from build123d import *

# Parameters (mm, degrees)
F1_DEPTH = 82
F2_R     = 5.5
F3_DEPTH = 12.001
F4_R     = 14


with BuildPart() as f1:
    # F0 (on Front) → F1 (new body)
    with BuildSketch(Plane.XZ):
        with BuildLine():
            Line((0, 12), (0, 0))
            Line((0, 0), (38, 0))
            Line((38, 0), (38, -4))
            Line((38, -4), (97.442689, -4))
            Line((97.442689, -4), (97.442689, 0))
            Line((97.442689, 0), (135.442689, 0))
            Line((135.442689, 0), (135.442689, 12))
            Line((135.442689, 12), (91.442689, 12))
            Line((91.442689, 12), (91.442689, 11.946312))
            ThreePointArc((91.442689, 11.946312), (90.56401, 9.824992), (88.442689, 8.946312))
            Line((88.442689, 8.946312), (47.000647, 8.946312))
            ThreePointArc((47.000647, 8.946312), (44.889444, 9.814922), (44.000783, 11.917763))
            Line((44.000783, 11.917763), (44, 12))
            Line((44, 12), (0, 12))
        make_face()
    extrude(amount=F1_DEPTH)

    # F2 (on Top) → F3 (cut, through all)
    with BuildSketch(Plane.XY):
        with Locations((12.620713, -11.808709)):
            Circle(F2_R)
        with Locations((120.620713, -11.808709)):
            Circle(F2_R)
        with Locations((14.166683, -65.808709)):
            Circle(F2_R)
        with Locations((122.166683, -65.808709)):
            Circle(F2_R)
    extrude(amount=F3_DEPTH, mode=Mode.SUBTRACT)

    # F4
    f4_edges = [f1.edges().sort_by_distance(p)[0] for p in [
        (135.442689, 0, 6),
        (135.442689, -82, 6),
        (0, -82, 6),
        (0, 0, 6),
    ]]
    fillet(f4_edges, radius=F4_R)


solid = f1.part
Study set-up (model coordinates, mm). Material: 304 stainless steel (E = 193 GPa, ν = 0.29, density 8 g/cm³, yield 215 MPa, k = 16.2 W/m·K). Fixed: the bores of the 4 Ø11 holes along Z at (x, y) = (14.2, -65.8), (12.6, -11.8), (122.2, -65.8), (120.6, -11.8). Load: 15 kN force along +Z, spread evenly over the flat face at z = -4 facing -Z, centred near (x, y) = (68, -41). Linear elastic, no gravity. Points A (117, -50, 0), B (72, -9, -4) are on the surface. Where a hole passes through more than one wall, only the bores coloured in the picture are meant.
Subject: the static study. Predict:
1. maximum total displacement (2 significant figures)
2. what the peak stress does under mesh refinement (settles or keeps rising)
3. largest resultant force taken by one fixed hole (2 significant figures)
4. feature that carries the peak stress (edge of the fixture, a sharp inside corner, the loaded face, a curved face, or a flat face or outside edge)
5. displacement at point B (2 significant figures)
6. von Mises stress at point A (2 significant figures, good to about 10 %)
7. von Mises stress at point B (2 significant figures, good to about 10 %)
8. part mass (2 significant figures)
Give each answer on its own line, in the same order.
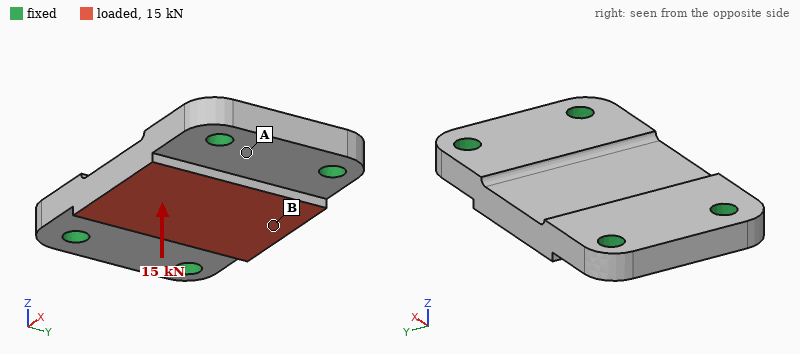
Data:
31 µm
keeps rising
6.0 kN
edge of the fixture
28 µm
23 MPa
50 MPa
1.1 kg
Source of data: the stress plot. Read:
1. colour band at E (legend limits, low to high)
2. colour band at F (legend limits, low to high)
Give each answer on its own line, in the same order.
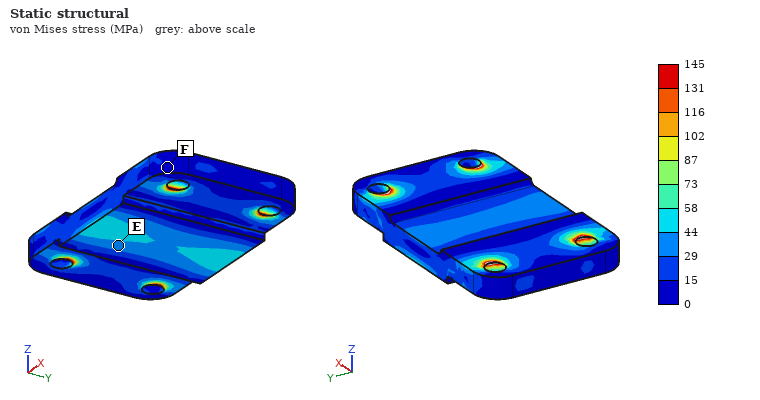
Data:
29 to 44 MPa
0 to 15 MPa
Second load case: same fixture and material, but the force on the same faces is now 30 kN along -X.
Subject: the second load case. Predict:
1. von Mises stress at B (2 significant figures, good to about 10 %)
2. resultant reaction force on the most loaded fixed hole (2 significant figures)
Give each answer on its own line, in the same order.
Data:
11 MPa
8.2 kN
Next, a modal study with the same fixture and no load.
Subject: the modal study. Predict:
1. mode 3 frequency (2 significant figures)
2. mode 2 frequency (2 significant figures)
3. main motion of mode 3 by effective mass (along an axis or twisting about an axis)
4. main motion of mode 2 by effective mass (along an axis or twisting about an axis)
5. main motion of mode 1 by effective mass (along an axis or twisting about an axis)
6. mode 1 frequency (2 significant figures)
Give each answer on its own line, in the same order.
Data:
12 kHz
6800 Hz
along Y
twisting about X
along Z
5200 Hz
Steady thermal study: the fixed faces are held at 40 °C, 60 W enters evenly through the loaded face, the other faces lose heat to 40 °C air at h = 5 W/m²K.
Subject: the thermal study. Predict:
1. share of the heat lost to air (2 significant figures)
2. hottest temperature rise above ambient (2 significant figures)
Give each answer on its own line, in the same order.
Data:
5.8 %
75 K
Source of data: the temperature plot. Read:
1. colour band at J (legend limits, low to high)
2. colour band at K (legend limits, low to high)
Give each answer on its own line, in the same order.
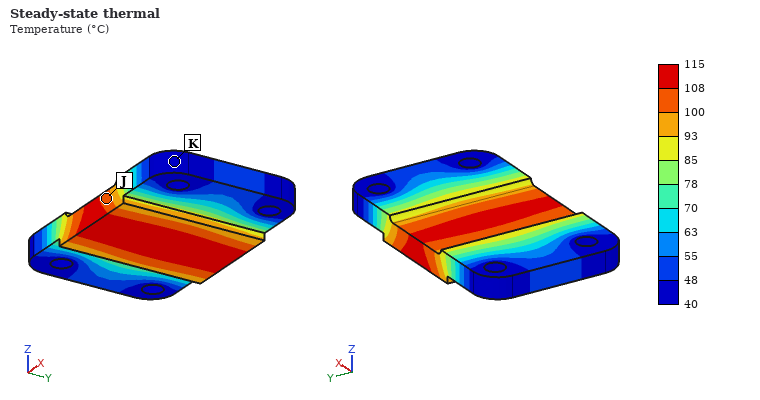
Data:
100 to 108 °C
40 to 48 °C
